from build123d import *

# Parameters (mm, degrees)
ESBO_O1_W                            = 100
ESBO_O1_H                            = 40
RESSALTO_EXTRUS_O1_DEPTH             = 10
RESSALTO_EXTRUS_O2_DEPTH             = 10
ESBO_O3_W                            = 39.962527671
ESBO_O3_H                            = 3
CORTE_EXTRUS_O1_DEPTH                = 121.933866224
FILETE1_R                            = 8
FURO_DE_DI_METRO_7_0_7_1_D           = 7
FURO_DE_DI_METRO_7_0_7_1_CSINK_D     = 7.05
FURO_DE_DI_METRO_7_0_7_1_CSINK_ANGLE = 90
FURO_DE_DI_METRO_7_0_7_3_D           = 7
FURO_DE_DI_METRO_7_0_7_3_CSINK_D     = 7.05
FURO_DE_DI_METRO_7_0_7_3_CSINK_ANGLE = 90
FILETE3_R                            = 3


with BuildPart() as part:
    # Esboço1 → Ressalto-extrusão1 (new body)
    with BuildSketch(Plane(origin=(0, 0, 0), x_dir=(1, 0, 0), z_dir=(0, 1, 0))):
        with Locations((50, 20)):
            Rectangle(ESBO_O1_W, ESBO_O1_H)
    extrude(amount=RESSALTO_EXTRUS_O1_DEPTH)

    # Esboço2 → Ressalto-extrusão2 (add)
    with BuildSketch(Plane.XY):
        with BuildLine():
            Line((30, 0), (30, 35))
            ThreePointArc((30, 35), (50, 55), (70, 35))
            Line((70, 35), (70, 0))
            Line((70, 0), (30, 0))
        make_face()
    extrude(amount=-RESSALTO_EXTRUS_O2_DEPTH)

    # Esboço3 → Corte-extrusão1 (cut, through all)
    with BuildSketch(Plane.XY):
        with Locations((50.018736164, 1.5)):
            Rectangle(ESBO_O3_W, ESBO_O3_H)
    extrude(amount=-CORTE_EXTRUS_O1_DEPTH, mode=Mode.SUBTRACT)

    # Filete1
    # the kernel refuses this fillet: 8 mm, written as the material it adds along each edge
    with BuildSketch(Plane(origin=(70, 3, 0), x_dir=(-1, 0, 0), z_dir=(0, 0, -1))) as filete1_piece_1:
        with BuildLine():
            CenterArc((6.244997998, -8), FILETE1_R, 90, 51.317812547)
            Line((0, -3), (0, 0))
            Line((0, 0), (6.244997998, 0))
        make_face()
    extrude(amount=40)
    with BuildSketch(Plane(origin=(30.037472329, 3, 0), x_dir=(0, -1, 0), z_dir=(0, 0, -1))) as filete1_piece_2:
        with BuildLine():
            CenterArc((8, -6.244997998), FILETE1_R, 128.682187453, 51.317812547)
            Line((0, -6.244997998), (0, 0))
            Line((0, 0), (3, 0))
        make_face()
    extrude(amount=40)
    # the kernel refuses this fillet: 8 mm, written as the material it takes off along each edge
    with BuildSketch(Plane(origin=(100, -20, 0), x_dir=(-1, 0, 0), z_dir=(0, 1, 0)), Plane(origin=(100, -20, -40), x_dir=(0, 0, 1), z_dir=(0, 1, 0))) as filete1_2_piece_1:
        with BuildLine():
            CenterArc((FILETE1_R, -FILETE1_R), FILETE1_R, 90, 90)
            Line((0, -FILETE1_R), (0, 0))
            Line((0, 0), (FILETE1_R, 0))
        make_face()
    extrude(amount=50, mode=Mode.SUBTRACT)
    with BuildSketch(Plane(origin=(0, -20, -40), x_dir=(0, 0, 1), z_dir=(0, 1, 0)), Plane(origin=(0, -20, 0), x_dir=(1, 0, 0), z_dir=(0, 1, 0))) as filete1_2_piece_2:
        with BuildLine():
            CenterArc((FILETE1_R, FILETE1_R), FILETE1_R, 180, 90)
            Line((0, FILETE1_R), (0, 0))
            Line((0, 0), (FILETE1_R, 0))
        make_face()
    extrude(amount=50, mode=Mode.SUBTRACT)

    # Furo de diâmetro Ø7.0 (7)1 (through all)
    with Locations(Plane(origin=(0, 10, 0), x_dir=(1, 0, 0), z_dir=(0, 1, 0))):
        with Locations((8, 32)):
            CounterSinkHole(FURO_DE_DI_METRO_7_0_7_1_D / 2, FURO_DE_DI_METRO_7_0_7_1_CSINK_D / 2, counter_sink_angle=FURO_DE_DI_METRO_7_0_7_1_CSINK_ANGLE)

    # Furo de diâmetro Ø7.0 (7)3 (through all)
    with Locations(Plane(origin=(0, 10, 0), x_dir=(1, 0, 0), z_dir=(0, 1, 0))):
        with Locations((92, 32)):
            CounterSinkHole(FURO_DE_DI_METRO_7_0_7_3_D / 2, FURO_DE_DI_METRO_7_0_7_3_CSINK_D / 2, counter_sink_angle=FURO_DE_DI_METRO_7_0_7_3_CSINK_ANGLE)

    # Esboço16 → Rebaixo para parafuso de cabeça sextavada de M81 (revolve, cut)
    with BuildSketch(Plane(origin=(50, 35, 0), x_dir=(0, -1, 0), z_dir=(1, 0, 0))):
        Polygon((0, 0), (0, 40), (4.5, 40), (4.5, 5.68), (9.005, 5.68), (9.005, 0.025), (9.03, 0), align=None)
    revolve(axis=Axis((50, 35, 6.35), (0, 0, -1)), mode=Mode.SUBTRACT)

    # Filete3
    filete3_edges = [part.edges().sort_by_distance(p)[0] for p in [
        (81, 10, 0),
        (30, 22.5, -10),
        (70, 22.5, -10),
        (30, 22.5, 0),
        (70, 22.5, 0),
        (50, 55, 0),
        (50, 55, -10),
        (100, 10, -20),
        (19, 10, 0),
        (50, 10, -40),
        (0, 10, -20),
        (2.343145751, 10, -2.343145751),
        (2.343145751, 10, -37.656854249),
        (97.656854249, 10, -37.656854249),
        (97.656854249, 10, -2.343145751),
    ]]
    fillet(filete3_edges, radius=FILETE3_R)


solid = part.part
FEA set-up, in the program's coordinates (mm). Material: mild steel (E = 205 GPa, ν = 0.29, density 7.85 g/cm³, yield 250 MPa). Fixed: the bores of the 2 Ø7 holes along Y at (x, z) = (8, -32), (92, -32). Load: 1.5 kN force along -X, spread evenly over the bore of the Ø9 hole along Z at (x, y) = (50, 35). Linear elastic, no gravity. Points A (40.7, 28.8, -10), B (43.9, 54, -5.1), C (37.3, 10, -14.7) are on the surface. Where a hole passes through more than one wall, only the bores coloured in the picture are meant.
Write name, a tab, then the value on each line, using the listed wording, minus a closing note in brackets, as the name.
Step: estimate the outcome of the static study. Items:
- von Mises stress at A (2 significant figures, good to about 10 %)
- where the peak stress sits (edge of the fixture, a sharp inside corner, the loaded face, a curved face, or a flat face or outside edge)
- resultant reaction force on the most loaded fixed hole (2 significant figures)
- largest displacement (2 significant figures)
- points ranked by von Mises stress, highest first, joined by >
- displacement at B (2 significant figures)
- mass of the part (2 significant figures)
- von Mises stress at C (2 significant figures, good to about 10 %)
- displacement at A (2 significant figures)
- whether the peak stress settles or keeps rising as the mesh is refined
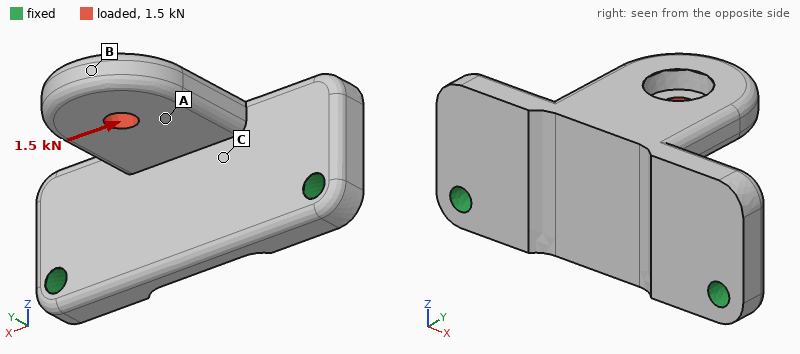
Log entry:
von Mises stress at A	17 MPa
where the peak stress sits	edge of the fixture
resultant reaction force on the most loaded fixed hole	1.1 kN
largest displacement	28 µm
points ranked by von Mises stress, highest first, joined by >	C > A > B
displacement at B	27 µm
mass of the part	380 g
von Mises stress at C	27 MPa
displacement at A	15 µm
whether the peak stress settles or keeps rising as the mesh is refined	keeps rising
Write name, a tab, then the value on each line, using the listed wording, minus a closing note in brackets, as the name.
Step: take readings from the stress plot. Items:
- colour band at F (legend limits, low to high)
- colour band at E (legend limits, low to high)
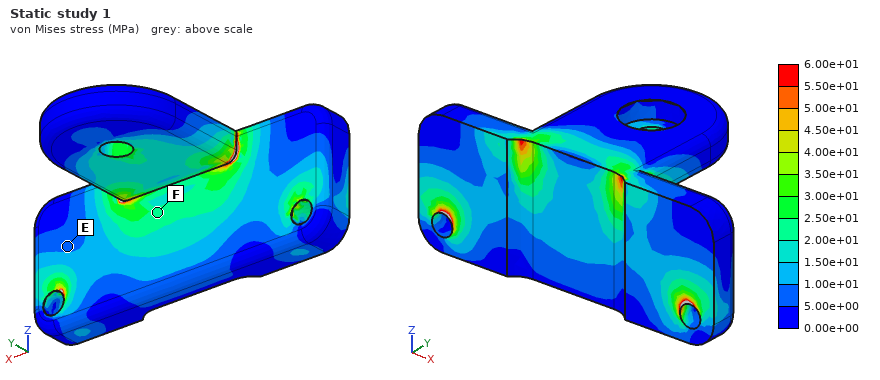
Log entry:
colour band at F	2.00e+01 to 2.50e+01 MPa
colour band at E	5.00e+00 to 1.00e+01 MPa
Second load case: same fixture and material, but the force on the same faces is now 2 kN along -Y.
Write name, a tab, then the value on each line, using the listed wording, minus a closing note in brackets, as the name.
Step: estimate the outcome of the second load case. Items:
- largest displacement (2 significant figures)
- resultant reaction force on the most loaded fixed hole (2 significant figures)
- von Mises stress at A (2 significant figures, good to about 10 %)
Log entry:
largest displacement	44 µm
resultant reaction force on the most loaded fixed hole	1.1 kN
von Mises stress at A	13 MPa
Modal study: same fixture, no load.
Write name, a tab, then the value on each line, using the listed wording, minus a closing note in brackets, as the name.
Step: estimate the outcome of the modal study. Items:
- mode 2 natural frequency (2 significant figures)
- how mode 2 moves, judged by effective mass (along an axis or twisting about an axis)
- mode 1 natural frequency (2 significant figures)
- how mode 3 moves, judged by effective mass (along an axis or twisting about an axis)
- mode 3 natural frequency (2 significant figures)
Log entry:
mode 2 natural frequency	4000 Hz
how mode 2 moves, judged by effective mass	along Y
mode 1 natural frequency	2100 Hz
how mode 3 moves, judged by effective mass	along X
mode 3 natural frequency	4200 Hz
